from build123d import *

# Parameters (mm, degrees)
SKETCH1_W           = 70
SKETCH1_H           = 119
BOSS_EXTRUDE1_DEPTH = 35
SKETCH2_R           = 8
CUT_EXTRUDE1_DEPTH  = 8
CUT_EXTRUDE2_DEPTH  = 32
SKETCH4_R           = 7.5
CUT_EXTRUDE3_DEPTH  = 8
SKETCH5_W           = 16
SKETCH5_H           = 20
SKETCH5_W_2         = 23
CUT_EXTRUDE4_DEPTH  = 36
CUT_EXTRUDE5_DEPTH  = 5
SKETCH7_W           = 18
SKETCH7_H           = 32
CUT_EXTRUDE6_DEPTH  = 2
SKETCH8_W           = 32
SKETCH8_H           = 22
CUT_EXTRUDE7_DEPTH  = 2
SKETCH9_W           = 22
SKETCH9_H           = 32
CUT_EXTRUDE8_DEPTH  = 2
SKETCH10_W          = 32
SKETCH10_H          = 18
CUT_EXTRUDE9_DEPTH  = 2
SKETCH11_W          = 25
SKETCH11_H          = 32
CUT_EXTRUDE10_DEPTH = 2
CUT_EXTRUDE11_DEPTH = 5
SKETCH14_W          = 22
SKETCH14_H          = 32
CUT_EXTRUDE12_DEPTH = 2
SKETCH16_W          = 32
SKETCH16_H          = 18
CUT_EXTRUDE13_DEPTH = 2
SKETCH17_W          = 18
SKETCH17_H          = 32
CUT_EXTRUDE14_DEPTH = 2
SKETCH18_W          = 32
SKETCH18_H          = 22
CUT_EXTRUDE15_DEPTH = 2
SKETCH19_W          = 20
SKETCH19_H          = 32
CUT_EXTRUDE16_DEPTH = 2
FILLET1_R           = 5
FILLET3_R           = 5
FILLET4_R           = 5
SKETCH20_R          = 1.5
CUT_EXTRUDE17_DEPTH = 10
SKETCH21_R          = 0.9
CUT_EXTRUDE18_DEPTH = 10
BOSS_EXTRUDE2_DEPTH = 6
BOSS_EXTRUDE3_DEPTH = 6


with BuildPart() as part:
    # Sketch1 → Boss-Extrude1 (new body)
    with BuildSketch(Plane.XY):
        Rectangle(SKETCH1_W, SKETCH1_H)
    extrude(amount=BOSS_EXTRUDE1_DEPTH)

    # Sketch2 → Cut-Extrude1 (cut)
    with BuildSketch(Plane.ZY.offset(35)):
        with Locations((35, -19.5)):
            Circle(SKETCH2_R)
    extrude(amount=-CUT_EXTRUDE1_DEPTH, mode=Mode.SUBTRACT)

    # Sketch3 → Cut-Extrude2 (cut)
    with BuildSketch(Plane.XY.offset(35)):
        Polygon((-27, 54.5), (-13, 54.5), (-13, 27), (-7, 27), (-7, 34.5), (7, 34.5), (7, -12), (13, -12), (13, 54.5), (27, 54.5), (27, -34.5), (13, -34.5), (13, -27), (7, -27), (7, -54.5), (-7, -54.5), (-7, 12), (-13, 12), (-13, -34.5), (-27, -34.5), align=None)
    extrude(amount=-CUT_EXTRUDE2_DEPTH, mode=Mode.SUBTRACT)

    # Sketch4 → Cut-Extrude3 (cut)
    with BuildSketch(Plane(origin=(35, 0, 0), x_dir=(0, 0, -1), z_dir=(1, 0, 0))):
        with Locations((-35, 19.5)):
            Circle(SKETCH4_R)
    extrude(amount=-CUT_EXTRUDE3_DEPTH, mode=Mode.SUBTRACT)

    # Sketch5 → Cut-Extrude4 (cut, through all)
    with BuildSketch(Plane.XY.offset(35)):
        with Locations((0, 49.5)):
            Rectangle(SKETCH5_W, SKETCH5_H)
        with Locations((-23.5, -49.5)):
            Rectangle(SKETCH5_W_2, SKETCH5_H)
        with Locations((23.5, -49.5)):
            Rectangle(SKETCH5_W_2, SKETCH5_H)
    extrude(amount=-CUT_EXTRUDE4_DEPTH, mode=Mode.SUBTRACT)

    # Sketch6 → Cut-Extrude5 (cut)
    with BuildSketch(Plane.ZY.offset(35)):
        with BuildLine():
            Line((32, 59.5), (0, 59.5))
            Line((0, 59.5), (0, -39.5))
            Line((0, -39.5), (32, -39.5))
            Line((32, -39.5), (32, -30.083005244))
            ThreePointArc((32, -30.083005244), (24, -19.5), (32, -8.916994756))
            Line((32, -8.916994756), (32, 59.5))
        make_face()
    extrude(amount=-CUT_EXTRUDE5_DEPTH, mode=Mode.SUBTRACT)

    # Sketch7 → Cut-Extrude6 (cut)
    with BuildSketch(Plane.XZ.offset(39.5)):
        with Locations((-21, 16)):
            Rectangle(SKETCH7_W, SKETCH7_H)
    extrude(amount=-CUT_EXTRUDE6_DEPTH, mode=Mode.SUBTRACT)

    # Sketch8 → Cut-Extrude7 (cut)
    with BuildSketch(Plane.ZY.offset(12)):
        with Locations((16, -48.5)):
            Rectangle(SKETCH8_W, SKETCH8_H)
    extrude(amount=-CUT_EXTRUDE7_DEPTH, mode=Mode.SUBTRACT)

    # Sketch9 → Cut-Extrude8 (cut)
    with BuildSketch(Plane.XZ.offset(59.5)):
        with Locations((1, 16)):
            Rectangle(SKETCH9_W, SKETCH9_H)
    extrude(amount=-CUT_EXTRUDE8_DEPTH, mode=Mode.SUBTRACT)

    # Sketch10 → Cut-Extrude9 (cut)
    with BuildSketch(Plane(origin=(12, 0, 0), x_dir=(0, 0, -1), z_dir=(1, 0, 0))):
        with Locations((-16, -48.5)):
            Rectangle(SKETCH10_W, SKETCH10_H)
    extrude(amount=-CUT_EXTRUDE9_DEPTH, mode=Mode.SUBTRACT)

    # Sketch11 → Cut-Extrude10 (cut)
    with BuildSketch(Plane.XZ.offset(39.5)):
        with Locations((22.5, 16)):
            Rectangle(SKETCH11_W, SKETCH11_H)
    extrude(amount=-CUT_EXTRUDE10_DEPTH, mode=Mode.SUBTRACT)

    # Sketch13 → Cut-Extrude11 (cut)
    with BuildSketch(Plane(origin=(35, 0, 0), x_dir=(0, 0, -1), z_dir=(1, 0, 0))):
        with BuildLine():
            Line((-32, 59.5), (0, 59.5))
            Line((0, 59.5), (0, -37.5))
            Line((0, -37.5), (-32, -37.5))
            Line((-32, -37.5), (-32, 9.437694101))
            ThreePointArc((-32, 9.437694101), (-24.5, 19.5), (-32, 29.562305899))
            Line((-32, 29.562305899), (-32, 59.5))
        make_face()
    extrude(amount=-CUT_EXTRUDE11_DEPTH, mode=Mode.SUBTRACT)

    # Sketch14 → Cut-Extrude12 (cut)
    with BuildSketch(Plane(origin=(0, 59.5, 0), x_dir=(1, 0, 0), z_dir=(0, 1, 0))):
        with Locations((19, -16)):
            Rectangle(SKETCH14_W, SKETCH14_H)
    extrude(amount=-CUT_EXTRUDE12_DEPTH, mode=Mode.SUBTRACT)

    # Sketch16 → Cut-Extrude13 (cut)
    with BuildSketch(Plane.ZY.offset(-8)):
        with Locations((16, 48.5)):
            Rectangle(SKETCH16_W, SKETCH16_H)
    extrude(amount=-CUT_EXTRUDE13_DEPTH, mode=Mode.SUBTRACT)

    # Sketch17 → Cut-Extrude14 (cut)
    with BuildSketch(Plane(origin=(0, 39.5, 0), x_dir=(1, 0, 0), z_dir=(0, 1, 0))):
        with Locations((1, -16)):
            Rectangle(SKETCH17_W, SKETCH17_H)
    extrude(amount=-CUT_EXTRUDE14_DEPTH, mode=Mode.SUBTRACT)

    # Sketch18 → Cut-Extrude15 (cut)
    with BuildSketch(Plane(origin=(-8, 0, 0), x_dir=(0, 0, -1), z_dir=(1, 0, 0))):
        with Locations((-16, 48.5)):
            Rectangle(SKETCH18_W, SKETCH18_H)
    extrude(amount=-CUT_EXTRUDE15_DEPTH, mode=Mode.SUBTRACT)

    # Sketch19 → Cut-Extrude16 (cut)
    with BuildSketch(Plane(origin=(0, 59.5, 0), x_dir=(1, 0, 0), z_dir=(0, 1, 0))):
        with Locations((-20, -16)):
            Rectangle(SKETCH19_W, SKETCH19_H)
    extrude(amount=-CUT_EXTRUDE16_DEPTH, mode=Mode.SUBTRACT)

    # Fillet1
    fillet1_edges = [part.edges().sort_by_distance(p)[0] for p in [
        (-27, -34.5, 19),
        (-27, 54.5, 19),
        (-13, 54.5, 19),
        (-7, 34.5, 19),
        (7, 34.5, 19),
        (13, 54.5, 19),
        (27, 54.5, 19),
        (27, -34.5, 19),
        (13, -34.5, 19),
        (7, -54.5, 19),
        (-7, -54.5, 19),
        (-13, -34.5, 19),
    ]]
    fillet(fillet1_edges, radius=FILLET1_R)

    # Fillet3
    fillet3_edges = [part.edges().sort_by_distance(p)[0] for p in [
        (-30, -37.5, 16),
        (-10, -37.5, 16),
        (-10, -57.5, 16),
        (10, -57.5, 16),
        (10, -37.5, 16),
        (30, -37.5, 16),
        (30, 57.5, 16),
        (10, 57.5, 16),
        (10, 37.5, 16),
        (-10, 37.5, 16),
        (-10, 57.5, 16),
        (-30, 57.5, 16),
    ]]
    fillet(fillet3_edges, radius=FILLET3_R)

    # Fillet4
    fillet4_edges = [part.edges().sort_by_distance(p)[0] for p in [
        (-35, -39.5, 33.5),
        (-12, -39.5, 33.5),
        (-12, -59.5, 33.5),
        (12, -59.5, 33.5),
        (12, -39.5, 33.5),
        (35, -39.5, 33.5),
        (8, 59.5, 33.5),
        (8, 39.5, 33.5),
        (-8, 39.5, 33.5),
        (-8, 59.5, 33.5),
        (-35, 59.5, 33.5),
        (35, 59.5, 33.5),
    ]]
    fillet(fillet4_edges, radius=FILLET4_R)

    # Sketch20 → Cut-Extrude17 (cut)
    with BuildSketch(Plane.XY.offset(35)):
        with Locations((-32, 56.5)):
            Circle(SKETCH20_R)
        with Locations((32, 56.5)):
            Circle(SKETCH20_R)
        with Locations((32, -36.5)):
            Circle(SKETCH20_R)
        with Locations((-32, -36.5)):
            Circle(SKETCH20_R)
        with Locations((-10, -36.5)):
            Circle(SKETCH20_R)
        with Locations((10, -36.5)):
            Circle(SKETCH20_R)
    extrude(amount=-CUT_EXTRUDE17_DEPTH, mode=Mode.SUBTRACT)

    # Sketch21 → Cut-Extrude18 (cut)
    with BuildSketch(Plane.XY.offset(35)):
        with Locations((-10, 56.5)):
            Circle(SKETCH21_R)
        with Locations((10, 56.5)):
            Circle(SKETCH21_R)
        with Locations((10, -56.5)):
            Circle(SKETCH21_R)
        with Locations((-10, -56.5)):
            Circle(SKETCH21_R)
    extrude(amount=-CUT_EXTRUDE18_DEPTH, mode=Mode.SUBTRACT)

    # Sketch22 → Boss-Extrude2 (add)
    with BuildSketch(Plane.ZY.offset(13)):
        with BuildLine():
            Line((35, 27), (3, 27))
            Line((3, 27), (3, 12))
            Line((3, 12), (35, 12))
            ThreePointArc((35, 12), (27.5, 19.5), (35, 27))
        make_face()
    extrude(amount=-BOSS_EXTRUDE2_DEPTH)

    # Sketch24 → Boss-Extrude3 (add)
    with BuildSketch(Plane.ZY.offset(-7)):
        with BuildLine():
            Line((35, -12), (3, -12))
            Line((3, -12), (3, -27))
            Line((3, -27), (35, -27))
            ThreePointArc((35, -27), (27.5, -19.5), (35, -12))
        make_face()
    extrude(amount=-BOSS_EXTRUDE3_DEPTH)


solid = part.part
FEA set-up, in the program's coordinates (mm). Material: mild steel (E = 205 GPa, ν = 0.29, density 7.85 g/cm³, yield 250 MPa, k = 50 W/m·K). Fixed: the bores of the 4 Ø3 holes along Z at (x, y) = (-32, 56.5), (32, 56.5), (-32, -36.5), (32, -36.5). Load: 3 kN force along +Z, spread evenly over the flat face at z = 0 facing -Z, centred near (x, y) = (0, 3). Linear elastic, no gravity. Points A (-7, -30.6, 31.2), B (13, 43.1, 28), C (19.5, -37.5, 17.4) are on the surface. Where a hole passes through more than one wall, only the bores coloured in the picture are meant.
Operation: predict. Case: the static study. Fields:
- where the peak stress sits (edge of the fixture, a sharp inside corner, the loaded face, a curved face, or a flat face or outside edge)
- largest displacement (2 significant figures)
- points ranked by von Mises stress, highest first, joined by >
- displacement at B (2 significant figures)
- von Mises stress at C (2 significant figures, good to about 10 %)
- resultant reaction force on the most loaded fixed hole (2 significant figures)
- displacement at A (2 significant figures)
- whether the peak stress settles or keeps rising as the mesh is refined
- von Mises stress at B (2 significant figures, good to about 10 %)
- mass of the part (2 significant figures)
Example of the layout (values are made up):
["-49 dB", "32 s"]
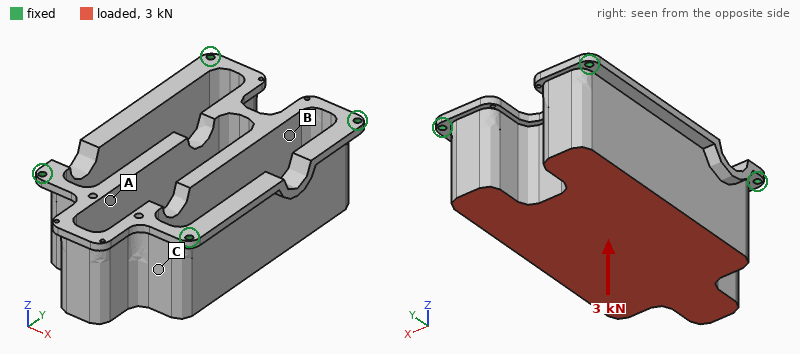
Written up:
["edge of the fixture", "8.4 µm", "C > B > A", "6.5 µm", "12 MPa", "1.0 kN", "6.3 µm", "keeps rising", "7.9 MPa", "660 g"]
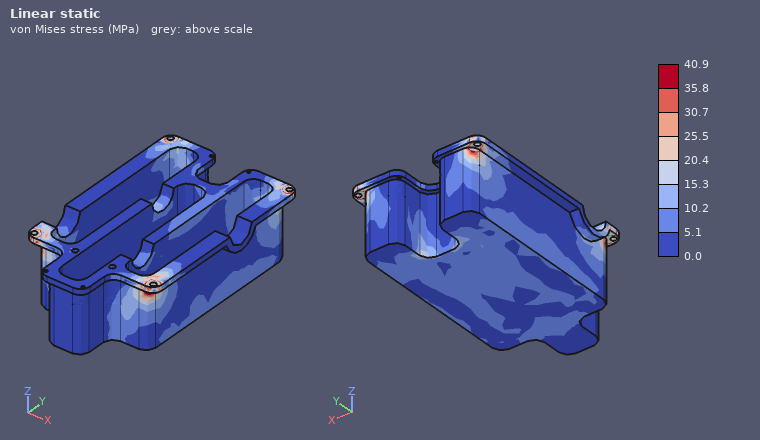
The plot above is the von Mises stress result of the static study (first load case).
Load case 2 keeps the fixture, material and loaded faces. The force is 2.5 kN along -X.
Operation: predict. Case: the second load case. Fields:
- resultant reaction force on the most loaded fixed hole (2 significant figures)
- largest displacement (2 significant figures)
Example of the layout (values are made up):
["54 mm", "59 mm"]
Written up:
["1.2 kN", "14 µm"]
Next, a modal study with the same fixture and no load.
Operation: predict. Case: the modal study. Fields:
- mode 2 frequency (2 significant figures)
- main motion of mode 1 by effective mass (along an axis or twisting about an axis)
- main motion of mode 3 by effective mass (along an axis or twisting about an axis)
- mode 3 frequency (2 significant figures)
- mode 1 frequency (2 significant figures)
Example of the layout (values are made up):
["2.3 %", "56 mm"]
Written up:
["3800 Hz", "along X", "along Z", "4200 Hz", "3300 Hz"]
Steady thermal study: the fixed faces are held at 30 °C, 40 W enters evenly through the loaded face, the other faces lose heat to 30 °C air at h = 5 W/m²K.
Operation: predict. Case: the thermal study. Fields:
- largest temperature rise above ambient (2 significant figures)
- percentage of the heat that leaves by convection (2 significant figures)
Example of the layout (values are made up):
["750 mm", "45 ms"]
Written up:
["61 K", "24 %"]
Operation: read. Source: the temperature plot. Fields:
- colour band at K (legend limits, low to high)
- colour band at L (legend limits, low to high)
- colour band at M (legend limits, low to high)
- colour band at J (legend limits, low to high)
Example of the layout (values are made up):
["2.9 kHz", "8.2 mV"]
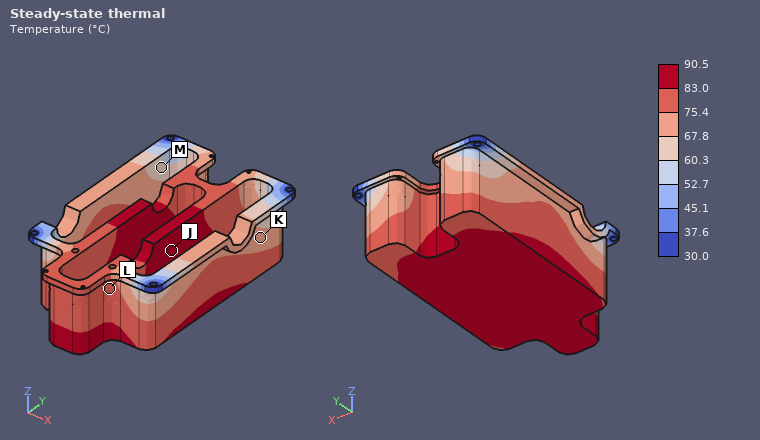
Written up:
["67.8 to 75.4 °C", "75.4 to 83.0 °C", "60.3 to 67.8 °C", "83.0 to 90.5 °C"]
